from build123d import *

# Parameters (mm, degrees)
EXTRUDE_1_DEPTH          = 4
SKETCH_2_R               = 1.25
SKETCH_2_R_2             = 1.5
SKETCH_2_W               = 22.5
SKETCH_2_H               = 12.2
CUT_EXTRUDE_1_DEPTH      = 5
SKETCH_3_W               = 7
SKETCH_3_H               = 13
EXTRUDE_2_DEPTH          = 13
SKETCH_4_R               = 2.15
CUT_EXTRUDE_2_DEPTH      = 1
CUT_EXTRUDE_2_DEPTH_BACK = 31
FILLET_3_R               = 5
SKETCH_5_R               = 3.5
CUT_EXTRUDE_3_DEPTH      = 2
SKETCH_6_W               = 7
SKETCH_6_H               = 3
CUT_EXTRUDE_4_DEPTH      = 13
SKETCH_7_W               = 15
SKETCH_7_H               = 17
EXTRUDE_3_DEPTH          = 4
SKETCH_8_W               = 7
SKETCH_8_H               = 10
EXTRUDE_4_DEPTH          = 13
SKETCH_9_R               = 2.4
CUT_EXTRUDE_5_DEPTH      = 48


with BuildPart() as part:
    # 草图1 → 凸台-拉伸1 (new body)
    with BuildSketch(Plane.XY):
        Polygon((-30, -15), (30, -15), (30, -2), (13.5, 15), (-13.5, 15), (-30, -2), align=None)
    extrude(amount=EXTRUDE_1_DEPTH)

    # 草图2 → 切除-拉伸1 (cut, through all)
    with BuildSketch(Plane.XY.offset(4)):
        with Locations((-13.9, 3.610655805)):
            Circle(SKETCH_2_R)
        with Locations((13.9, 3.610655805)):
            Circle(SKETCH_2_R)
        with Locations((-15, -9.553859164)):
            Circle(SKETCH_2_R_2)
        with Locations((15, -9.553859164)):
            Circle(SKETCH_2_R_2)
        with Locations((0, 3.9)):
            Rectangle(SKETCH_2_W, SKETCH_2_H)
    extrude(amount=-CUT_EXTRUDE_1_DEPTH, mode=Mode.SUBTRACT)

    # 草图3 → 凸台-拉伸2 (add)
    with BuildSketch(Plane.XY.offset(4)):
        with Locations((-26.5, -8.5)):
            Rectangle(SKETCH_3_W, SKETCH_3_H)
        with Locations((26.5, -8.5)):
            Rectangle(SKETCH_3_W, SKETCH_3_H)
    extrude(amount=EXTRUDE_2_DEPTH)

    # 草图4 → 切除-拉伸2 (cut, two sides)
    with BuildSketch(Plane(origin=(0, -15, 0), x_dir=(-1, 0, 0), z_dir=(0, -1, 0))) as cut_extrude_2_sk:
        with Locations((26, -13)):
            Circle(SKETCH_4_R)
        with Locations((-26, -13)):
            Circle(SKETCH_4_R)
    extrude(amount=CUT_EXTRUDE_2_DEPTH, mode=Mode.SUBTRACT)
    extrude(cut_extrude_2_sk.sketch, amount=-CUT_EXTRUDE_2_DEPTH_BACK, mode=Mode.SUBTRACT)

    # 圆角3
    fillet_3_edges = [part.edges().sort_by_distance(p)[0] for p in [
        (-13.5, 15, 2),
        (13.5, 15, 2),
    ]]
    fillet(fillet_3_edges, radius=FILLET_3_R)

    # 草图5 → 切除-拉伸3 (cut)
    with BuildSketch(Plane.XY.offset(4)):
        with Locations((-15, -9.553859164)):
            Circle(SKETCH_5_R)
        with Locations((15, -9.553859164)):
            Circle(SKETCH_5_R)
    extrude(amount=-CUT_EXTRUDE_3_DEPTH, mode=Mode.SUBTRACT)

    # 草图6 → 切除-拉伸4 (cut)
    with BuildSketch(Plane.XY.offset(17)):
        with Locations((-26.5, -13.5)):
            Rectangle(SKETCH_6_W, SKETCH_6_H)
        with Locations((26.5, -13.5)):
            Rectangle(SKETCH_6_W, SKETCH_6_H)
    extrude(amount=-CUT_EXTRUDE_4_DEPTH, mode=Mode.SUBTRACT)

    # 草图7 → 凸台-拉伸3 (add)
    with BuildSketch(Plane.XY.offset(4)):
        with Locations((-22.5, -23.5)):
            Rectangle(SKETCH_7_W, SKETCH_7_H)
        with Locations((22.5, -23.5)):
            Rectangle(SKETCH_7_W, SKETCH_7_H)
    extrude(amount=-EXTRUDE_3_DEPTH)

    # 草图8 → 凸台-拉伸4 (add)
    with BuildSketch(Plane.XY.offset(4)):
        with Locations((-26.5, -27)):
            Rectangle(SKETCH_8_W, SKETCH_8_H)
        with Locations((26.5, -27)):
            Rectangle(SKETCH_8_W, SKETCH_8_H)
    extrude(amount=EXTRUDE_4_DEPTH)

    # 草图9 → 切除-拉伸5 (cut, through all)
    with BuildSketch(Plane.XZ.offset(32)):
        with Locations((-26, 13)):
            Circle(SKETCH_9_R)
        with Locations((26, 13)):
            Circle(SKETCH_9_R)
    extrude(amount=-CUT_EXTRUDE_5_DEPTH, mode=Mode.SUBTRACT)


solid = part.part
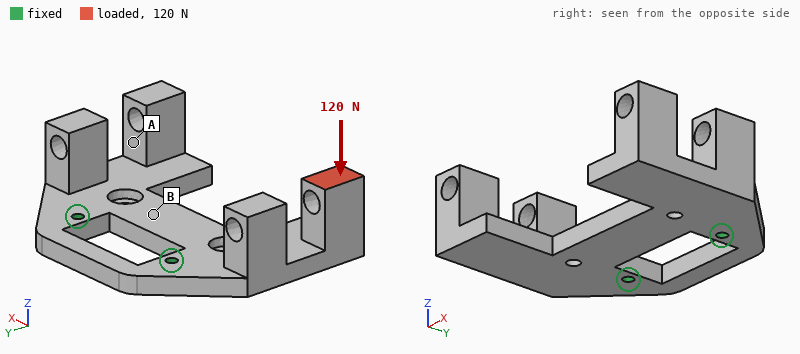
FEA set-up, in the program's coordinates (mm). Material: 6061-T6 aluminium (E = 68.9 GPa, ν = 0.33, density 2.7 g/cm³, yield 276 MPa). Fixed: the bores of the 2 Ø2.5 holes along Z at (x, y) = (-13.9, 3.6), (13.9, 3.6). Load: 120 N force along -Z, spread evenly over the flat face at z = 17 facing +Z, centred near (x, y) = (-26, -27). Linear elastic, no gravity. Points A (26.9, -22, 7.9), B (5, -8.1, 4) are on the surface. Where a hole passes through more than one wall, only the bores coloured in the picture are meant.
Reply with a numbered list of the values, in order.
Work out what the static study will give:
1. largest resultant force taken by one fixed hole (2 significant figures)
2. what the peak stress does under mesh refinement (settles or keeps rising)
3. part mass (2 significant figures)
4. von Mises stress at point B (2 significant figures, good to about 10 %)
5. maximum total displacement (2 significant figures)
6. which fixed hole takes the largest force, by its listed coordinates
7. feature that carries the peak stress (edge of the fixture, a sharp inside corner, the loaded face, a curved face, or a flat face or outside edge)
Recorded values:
1. 140 N
2. keeps rising
3. 26 g
4. 23 MPa
5. 0.33 mm
6. (-13.9, 3.6)
7. edge of the fixture
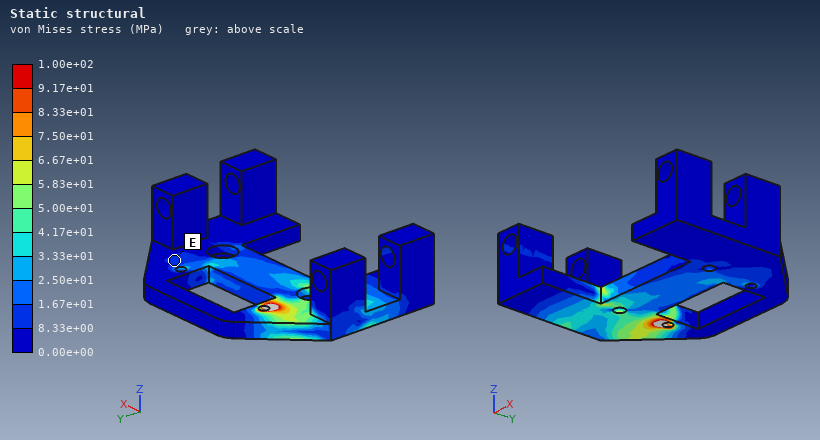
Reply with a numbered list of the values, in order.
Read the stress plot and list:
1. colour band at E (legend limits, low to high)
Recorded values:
1. 8.33e+00 to 1.67e+01 MPa
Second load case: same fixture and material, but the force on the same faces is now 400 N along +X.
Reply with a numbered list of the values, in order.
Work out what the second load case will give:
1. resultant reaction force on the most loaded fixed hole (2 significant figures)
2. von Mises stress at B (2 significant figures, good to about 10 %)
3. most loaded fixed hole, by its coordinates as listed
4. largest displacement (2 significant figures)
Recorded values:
1. 470 N
2. 25 MPa
3. (13.9, 3.6)
4. 0.51 mm
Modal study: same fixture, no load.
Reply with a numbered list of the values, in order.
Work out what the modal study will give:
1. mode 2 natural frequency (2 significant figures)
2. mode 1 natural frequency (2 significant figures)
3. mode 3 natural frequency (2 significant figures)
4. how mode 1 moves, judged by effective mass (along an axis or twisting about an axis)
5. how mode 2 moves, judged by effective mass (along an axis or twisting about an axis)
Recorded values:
1. 1800 Hz
2. 1600 Hz
3. 4200 Hz
4. along Z
5. twisting about Y
